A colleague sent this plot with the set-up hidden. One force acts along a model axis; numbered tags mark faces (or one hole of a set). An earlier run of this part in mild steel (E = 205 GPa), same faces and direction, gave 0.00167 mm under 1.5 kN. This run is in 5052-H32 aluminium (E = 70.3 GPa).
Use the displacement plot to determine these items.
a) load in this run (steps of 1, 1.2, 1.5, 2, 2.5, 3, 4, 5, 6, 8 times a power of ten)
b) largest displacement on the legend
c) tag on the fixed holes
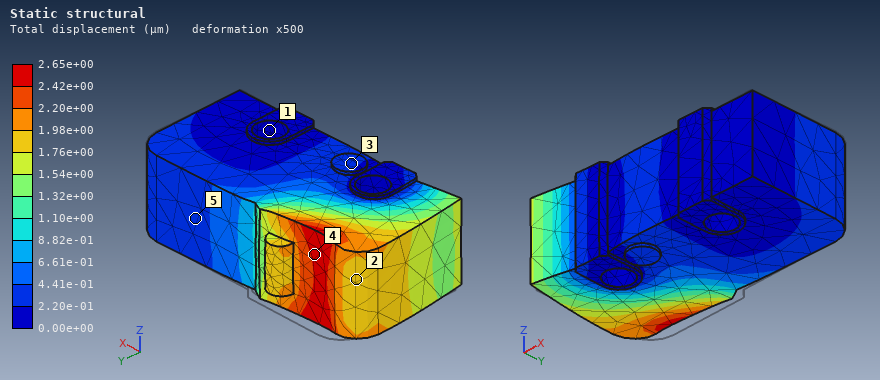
800 N
2.65e+00 µm
1
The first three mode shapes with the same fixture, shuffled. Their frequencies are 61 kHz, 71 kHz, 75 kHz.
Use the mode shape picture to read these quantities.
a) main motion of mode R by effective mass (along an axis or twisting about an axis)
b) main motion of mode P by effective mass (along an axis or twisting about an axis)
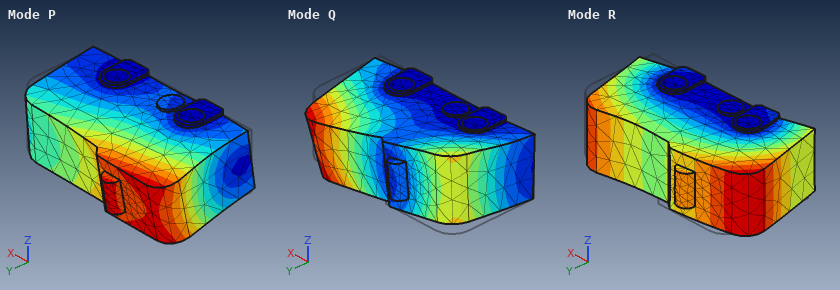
along X
along Z
